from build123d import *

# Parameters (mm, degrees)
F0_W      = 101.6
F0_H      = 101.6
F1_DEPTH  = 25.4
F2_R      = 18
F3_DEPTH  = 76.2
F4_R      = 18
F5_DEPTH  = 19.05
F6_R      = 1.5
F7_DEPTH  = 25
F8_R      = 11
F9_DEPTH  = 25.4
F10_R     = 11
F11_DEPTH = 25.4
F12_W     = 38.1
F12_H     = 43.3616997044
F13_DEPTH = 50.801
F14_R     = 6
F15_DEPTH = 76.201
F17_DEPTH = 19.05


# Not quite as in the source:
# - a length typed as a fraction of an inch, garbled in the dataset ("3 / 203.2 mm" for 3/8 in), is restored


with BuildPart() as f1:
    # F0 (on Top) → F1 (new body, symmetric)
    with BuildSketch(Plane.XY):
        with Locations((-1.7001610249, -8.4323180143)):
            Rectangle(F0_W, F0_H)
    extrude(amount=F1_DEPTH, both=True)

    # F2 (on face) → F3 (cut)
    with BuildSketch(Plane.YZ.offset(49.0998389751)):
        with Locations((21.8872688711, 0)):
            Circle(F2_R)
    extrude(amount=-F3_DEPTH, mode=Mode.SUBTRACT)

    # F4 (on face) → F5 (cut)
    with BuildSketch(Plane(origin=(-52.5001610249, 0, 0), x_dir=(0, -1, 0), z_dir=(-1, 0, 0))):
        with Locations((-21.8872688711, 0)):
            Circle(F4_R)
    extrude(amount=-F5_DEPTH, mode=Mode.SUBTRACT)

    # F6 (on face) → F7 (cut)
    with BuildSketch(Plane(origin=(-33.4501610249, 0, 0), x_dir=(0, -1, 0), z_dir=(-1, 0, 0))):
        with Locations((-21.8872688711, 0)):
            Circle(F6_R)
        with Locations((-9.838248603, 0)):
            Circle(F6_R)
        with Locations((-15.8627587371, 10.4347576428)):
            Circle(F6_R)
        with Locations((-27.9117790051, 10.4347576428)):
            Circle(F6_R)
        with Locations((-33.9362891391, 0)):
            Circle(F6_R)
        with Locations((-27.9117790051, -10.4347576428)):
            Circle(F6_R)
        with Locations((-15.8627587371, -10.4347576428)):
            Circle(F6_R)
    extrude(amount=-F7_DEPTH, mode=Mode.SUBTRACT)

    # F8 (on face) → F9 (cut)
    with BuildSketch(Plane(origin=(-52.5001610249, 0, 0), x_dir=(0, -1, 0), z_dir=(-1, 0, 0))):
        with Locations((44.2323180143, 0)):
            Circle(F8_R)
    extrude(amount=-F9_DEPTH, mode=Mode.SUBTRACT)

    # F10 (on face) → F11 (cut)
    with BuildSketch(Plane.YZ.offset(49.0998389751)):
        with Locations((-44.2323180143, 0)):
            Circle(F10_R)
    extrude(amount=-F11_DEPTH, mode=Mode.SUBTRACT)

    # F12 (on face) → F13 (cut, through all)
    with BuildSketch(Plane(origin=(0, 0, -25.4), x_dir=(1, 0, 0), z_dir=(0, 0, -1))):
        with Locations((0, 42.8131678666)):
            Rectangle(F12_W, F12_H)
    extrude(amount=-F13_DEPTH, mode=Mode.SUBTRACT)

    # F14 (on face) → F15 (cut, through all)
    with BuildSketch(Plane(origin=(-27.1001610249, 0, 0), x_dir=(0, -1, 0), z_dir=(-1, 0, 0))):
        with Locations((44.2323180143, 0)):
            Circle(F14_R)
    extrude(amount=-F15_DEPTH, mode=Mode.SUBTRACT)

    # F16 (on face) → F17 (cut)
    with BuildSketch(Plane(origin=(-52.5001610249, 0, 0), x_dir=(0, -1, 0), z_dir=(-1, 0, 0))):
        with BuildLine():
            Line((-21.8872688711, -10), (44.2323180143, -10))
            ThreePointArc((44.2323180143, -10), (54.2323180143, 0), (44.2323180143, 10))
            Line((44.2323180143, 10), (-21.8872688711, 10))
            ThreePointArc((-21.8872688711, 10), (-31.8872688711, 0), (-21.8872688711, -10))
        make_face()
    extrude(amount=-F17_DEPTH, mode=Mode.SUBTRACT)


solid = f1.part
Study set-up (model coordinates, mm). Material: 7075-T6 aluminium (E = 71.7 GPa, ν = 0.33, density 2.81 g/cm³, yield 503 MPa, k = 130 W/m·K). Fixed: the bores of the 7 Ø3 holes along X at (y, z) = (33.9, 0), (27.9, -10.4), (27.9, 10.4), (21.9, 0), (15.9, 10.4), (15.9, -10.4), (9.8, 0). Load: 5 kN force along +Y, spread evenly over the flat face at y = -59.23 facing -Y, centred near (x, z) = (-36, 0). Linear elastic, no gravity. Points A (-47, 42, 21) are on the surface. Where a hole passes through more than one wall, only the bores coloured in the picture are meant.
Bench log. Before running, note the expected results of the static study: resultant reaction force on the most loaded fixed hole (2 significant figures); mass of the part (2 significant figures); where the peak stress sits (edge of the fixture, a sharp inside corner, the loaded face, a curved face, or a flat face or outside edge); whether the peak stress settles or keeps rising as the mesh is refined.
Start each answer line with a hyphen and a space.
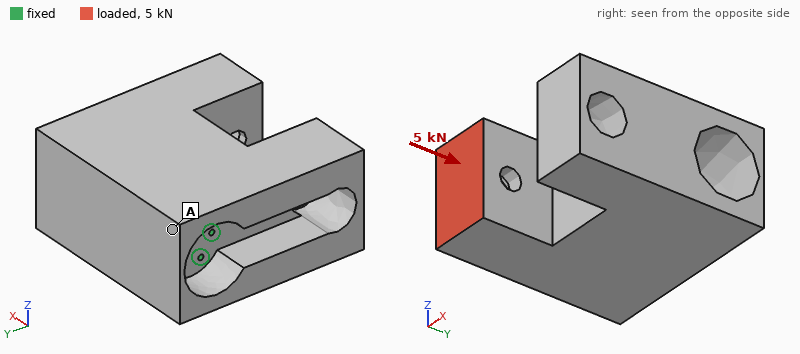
- 1.3 kN
- 890 g
- edge of the fixture
- keeps rising
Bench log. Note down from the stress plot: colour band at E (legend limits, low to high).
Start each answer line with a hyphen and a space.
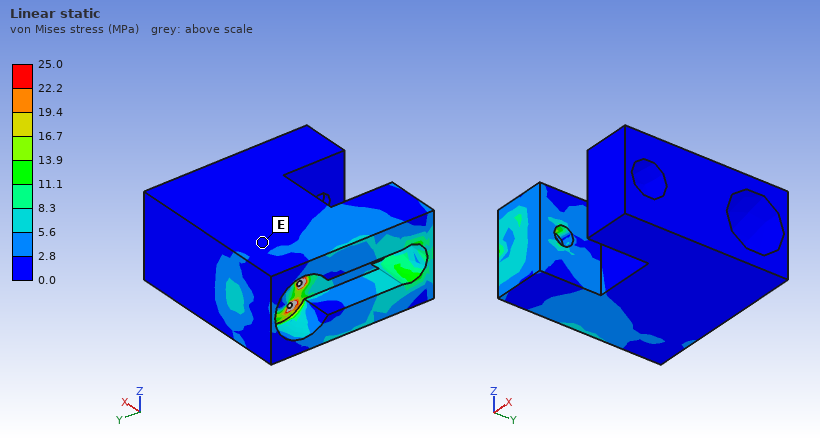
- 0.0 to 2.8 MPa
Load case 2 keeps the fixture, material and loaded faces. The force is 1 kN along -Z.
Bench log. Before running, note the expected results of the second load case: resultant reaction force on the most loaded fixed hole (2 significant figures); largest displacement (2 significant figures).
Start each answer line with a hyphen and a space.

- 1.2 kN
- 31 µm
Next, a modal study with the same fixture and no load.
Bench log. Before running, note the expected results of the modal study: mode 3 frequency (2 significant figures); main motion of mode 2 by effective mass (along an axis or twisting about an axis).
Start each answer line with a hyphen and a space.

- 2600 Hz
- along Z
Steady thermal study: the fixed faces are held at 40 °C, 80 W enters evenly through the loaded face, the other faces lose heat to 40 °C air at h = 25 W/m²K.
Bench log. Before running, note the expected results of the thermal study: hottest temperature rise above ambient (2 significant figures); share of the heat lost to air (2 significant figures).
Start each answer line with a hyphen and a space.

- 41 K
- 21 %
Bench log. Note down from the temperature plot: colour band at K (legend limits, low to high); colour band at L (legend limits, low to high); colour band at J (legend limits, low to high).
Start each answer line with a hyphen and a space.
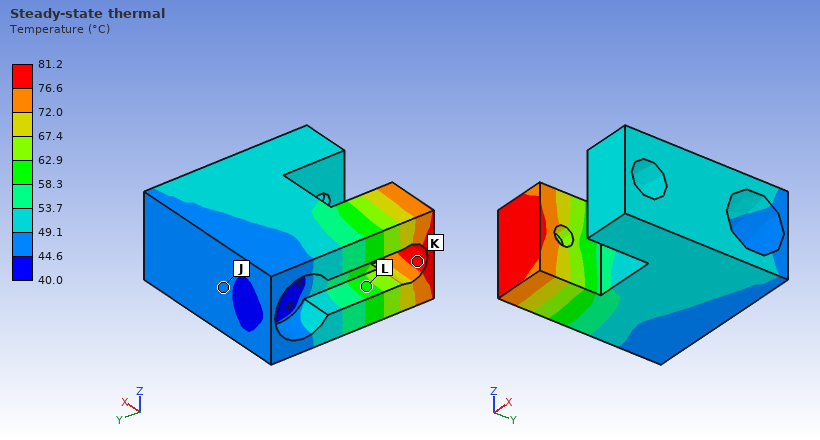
- 76.6 to 81.2 °C
- 58.3 to 62.9 °C
- 44.6 to 49.1 °C
